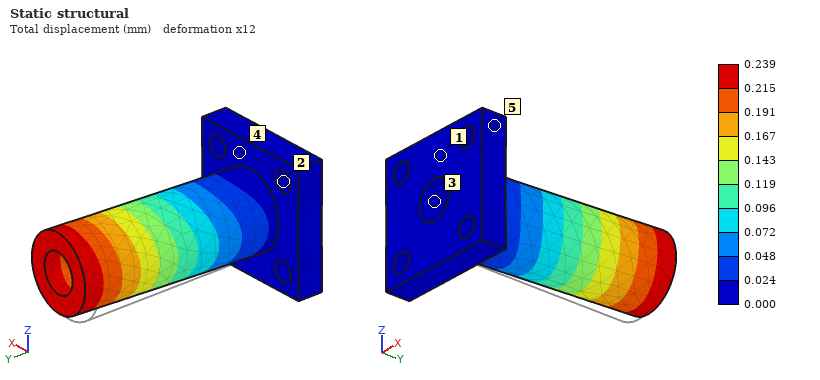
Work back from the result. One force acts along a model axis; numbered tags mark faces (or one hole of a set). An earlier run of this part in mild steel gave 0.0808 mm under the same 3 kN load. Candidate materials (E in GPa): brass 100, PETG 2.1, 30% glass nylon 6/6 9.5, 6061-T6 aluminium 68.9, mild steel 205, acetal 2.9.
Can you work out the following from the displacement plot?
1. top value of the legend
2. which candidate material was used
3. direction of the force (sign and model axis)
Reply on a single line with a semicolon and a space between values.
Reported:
0.239 mm; 6061-T6 aluminium; +X
